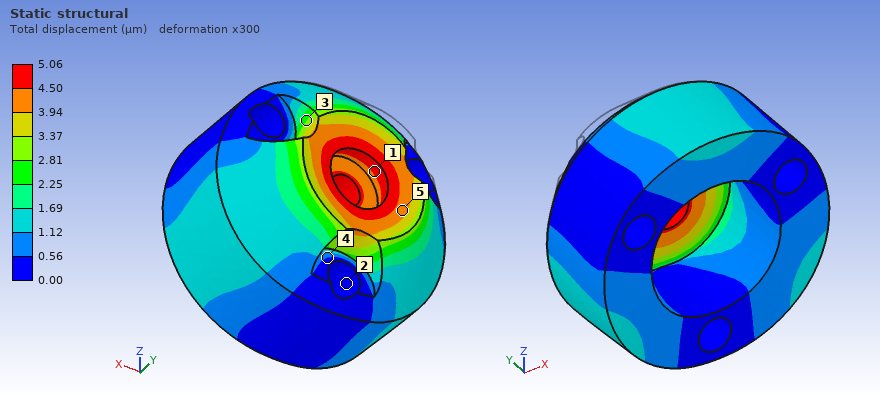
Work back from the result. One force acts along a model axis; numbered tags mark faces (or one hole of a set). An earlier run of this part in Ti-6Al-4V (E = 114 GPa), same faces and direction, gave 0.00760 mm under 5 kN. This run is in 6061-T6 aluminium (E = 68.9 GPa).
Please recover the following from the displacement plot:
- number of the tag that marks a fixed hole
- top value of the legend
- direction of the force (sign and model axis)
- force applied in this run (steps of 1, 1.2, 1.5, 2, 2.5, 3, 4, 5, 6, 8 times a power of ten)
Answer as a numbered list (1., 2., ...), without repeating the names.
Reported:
1. 2
2. 5.06 µm
3. -Y
4. 2 kN
